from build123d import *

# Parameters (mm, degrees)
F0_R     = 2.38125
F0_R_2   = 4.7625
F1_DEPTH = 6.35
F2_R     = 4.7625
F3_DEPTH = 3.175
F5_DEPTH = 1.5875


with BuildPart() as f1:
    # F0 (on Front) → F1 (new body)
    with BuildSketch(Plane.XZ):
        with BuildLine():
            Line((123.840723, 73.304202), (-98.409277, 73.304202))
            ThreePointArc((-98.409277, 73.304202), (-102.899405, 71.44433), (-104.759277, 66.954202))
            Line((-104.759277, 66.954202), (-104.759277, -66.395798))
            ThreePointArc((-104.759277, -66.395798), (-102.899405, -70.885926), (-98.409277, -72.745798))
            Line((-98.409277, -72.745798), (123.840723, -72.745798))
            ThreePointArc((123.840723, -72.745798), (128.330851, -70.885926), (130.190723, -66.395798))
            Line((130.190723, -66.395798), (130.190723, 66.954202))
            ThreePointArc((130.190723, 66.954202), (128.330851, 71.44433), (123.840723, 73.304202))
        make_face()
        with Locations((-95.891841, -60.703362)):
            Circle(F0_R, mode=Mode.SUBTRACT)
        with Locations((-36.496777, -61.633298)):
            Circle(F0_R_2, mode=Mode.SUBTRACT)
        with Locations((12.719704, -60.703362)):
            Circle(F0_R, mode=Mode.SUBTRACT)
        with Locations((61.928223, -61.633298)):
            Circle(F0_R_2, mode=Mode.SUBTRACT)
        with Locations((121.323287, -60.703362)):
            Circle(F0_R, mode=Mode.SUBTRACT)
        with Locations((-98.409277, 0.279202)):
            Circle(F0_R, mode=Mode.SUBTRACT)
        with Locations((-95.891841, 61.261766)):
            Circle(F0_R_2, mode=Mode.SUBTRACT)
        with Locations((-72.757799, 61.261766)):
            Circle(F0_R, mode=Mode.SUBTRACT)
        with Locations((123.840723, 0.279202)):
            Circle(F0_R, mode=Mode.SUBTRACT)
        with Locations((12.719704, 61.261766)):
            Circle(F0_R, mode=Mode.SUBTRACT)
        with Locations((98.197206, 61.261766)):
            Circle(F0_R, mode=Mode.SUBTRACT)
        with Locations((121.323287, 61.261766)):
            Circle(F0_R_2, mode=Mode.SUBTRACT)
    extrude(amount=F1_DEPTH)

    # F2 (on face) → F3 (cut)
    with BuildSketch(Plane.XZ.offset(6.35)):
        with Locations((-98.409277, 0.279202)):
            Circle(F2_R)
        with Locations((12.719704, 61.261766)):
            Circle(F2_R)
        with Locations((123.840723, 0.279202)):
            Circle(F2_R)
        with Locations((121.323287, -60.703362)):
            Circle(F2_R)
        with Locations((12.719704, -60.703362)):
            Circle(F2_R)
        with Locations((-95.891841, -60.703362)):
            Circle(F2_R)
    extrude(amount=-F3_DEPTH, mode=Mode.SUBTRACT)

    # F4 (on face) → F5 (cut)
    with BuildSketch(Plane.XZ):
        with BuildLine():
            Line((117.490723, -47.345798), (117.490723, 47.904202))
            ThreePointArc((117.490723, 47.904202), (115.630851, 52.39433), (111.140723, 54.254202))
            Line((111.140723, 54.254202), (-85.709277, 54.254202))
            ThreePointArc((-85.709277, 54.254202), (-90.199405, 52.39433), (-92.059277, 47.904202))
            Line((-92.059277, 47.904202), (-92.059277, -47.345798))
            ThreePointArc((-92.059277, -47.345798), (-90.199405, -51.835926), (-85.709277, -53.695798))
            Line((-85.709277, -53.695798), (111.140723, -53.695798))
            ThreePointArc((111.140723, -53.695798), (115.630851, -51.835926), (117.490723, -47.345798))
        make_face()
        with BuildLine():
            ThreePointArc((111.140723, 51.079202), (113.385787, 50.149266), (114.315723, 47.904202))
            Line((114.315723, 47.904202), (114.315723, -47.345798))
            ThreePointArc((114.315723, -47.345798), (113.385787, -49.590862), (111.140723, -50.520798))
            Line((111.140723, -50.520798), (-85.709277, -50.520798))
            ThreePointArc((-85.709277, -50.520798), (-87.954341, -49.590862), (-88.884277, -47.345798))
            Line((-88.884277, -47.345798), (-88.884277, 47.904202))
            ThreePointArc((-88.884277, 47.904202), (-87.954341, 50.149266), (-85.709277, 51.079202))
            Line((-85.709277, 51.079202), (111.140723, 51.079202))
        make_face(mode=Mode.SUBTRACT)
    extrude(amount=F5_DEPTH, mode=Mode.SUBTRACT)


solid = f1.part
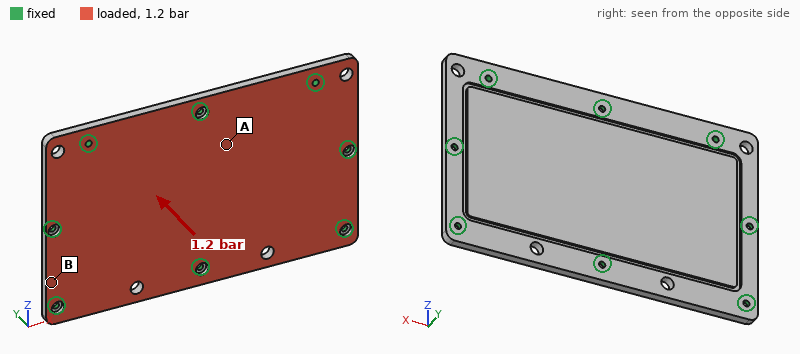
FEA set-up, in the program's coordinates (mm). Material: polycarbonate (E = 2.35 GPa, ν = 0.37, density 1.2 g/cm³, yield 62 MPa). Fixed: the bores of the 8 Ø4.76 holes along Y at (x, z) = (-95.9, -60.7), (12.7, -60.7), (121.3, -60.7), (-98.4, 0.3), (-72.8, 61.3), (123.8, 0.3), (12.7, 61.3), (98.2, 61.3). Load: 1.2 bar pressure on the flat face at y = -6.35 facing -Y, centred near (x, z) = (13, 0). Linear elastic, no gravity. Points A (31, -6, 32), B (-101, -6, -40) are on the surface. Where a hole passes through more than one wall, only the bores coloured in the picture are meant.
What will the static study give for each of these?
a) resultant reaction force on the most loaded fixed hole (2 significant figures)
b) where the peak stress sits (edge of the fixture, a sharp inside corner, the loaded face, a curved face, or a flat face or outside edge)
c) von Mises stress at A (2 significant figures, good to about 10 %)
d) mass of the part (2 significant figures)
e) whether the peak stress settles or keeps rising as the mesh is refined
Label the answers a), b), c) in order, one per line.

a) 1.1 kN
b) edge of the fixture
c) 11 MPa
d) 250 g
e) keeps rising
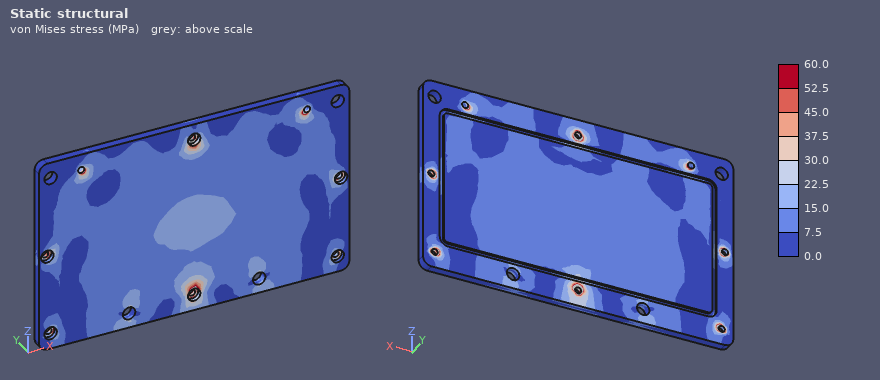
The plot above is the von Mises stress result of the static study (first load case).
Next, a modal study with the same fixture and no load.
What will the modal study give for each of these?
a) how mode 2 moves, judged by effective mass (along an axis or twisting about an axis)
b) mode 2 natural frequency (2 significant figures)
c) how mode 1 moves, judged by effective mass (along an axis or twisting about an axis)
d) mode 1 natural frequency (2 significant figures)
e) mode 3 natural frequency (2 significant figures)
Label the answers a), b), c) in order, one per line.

a) twisting about Z
b) 520 Hz
c) along Y
d) 430 Hz
e) 760 Hz
